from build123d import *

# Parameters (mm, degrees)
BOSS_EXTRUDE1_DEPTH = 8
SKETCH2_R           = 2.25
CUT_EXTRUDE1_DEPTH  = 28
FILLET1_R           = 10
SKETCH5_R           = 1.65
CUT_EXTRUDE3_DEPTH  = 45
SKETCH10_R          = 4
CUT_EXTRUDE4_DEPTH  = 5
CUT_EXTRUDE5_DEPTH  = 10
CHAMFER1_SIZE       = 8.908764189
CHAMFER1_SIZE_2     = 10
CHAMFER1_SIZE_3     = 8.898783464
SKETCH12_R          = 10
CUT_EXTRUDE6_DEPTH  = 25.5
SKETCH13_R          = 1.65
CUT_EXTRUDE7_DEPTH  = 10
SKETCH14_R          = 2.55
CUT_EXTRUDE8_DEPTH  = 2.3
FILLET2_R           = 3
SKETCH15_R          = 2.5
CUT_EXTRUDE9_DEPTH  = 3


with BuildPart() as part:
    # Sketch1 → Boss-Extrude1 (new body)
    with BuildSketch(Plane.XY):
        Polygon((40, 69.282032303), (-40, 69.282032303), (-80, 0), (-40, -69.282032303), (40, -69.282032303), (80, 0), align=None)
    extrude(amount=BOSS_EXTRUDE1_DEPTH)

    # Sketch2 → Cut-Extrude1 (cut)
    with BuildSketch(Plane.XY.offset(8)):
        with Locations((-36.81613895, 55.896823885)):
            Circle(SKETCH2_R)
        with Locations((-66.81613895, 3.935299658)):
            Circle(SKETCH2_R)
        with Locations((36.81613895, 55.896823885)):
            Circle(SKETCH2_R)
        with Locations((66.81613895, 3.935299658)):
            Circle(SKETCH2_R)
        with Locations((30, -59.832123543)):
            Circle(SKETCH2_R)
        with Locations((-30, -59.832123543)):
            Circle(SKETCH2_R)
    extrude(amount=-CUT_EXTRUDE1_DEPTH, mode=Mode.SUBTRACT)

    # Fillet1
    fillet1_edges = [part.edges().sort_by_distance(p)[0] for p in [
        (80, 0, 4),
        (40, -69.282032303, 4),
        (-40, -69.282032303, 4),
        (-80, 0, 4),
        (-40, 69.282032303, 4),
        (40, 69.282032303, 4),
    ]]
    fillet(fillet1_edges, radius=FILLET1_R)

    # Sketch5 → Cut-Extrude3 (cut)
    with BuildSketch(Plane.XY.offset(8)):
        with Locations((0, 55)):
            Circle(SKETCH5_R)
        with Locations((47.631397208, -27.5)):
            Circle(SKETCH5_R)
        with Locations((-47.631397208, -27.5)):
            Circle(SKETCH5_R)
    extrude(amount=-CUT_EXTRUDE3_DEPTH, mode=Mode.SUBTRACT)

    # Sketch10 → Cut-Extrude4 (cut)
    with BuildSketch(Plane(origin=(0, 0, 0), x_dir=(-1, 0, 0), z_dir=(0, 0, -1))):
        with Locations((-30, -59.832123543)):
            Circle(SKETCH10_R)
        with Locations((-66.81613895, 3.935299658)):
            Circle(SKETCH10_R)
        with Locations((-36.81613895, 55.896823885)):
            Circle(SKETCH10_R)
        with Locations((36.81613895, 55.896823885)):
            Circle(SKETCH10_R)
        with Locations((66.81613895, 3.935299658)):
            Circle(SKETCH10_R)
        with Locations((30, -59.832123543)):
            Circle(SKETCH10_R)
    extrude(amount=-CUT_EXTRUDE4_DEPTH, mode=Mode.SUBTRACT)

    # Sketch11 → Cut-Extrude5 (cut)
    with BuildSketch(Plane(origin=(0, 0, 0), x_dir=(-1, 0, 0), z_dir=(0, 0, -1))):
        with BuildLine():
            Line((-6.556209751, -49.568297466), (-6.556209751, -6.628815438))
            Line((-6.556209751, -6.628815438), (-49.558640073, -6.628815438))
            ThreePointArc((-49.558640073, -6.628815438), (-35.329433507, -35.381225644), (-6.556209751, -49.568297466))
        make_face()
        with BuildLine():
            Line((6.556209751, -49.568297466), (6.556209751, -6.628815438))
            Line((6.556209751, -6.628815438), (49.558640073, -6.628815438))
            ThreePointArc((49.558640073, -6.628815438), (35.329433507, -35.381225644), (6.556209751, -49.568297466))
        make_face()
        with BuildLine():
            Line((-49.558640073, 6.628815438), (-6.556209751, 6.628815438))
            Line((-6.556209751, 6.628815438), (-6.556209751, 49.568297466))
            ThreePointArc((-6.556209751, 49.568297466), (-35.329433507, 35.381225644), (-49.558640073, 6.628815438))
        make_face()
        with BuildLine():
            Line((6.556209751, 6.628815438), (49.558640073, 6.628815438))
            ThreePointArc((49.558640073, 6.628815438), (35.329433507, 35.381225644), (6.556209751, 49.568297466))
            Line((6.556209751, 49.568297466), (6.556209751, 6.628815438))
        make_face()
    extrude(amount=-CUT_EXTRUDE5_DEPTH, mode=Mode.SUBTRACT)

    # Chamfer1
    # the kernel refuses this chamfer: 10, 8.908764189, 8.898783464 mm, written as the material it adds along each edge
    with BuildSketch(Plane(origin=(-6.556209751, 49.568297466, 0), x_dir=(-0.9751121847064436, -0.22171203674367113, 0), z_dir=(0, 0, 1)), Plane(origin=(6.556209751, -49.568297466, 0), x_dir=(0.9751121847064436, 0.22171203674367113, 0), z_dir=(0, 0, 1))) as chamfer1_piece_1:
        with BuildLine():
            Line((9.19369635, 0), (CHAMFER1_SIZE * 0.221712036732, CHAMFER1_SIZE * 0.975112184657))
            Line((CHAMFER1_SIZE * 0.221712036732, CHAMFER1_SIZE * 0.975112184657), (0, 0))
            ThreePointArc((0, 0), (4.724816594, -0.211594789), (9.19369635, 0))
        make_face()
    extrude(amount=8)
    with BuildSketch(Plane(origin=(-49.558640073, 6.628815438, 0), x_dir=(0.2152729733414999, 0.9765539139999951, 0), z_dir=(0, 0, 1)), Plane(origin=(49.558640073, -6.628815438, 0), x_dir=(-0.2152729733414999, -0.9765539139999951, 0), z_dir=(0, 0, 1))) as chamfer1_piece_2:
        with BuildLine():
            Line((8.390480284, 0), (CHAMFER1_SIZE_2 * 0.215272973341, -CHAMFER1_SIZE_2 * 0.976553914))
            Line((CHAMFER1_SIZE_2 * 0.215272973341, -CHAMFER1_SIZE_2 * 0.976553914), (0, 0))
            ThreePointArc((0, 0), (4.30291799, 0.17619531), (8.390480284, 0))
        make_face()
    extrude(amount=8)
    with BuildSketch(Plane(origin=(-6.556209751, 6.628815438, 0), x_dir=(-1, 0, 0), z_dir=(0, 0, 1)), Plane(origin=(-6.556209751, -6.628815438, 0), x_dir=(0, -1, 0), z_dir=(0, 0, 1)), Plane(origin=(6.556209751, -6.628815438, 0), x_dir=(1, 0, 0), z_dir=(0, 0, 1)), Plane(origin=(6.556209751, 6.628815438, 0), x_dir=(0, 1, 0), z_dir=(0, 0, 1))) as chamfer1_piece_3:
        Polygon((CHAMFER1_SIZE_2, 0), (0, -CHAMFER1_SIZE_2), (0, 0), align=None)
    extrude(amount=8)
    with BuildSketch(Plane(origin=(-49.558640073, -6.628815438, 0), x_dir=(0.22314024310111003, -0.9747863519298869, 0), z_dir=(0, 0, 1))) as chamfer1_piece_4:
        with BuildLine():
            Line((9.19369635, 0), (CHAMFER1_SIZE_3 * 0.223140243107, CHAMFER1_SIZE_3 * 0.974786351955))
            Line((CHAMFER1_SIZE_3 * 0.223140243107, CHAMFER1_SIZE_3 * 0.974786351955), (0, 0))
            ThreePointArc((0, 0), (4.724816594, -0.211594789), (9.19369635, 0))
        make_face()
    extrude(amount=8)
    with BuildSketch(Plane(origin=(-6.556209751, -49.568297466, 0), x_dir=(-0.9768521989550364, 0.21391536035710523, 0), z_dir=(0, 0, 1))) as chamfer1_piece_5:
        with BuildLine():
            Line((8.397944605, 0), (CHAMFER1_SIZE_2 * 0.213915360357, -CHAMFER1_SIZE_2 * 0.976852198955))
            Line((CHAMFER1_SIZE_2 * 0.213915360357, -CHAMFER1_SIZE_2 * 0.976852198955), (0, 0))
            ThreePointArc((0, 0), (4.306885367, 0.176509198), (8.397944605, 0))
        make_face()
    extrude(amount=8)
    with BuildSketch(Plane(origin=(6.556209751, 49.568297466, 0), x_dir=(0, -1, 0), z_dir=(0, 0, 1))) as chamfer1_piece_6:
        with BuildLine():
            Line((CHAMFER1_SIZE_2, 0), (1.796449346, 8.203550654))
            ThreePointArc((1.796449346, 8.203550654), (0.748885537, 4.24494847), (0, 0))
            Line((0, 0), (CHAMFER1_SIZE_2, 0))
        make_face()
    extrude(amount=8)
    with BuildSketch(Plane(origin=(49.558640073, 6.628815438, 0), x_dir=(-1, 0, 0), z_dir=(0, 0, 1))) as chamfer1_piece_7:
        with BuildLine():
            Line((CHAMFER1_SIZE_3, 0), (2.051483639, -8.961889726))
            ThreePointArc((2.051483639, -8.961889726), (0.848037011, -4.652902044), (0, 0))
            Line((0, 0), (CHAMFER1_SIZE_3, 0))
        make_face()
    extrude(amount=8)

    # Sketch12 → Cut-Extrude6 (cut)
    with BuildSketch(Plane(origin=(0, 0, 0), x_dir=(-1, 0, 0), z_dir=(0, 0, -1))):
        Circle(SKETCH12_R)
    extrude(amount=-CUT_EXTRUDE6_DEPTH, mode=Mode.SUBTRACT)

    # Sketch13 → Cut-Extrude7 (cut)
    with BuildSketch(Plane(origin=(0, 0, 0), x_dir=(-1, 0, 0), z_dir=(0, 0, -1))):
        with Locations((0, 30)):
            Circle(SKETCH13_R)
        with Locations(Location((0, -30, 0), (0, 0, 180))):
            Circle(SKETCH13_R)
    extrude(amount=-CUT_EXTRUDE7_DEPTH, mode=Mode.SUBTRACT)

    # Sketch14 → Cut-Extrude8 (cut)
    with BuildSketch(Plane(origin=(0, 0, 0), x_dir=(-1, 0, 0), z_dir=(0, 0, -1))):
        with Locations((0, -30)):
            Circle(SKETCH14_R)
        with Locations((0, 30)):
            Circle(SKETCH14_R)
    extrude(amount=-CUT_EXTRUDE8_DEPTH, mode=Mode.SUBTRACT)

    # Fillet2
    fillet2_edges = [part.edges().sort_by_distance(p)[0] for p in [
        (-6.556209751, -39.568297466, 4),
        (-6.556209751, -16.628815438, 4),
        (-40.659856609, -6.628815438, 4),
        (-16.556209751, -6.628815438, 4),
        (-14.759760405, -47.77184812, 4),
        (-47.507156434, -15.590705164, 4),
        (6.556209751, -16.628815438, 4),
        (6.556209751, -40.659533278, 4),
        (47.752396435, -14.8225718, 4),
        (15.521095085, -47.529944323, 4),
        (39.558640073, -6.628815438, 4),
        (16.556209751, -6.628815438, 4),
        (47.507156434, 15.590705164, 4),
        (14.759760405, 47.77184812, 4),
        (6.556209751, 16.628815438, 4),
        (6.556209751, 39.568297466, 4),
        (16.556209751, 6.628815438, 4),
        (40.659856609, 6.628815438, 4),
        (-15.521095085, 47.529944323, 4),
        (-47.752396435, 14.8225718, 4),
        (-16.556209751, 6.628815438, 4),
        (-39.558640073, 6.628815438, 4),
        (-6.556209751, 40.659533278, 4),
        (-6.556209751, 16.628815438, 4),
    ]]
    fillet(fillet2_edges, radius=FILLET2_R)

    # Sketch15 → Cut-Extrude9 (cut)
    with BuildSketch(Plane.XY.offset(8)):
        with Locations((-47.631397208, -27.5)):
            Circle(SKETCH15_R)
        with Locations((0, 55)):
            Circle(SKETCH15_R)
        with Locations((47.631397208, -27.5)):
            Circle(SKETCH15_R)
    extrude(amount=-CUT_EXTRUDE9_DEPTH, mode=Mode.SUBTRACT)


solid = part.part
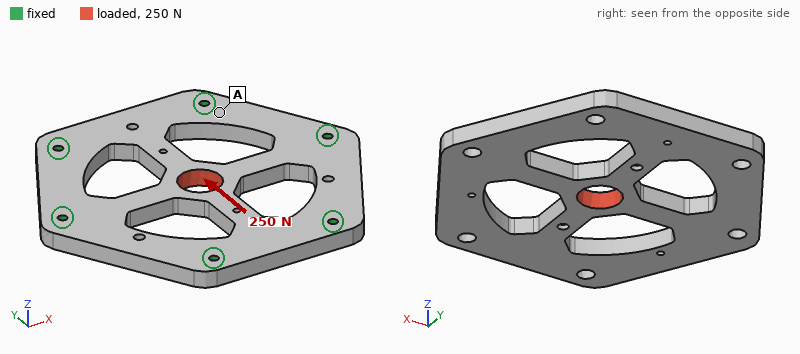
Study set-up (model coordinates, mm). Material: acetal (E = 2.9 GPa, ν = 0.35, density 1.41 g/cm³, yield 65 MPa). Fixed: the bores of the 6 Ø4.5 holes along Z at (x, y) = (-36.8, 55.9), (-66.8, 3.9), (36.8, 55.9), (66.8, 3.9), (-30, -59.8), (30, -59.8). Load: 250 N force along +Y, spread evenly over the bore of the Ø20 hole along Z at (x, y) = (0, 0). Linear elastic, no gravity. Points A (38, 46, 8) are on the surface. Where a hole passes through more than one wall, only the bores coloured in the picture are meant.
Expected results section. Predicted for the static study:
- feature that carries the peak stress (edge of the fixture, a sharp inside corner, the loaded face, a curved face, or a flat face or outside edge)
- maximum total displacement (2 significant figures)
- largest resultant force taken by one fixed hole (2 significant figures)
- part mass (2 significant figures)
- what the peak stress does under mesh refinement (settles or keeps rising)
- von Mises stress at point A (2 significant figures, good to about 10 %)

edge of the fixture
36 µm
57 N
130 g
keeps rising
0.34 MPa
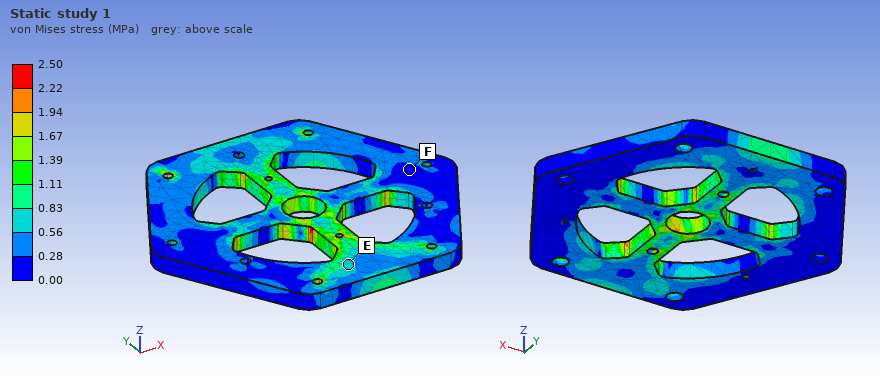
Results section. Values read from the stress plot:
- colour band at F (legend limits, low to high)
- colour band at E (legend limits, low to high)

0.00 to 0.28 MPa
0.56 to 0.83 MPa
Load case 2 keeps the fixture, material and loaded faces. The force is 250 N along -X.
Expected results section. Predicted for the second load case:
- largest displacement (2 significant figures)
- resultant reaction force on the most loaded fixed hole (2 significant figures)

28 µm
87 N
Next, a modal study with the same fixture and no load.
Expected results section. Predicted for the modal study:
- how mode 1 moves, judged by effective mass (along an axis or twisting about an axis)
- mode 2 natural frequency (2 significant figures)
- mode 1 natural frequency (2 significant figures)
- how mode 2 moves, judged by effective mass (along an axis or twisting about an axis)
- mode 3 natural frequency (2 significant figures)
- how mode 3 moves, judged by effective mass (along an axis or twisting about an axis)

along Z
1400 Hz
750 Hz
twisting about X
1500 Hz
twisting about Y
